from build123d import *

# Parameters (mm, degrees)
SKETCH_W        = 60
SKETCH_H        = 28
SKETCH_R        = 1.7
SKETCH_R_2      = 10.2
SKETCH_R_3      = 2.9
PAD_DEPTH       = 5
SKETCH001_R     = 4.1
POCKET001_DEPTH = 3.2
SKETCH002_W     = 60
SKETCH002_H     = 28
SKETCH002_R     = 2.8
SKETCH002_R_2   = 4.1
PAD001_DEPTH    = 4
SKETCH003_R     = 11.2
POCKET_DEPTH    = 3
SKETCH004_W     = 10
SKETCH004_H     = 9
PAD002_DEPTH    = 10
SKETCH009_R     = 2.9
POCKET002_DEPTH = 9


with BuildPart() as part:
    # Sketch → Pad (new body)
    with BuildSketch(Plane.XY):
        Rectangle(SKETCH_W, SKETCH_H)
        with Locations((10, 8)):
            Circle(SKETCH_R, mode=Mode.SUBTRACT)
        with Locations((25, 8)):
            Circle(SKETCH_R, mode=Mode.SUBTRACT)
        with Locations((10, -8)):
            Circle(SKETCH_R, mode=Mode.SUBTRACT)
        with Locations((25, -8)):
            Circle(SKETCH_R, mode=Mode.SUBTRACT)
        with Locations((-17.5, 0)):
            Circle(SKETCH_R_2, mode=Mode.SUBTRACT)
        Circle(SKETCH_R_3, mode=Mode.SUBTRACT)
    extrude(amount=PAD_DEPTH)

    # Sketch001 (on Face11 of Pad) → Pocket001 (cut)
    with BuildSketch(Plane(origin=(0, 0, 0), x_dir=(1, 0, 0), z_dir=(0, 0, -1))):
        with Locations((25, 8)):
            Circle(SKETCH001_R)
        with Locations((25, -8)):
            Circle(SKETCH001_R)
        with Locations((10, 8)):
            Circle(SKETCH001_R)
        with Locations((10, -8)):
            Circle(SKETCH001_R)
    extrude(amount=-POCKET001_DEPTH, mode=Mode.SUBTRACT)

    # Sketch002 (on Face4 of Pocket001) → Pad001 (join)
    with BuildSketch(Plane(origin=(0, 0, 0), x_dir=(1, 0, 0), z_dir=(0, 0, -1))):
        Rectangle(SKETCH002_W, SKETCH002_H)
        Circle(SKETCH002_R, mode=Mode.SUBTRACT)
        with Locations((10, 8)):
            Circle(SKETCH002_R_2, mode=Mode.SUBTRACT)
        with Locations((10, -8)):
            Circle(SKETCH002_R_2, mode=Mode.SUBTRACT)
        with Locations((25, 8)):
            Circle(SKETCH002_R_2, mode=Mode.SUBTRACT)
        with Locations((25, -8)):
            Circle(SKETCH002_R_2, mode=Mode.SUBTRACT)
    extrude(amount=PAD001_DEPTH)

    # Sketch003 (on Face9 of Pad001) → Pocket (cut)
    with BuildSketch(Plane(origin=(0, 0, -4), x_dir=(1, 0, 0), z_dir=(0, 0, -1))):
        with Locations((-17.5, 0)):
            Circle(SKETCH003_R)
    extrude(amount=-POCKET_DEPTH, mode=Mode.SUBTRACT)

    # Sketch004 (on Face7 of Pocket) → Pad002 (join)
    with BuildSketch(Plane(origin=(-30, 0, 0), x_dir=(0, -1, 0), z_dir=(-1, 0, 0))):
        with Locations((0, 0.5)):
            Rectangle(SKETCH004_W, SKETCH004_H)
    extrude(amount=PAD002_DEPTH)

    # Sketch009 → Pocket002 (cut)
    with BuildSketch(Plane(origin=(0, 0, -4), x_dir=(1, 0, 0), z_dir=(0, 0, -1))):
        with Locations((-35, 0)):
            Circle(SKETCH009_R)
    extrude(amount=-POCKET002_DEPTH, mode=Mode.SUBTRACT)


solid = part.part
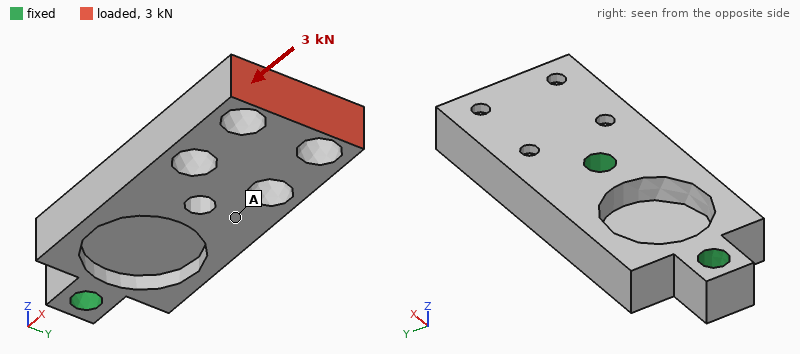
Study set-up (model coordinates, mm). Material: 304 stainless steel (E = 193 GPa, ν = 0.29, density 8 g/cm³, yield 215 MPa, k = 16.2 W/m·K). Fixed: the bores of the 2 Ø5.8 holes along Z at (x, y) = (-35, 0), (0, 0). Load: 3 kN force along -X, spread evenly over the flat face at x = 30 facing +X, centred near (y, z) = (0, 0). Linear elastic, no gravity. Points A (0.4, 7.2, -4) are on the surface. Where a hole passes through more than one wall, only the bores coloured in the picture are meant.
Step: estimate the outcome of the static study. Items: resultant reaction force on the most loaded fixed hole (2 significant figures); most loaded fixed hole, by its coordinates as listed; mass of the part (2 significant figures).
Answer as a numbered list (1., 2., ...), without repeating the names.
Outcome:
1. 2.7 kN
2. (0, 0)
3. 89 g
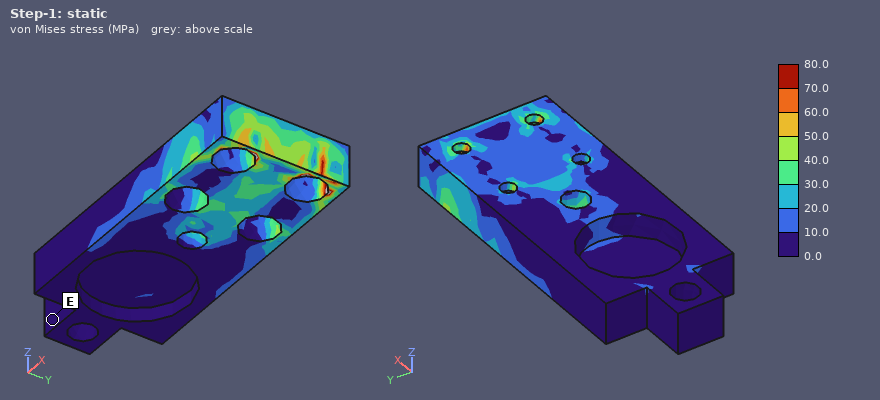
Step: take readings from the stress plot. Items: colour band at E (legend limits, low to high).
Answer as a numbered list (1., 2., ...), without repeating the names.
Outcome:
1. 0.0 to 10.0 MPa
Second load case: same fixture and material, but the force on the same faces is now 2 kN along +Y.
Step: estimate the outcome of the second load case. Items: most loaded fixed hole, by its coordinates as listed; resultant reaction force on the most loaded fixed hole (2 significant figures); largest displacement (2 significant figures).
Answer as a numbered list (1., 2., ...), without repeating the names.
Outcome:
1. (0, 0)
2. 3.0 kN
3. 36 µm
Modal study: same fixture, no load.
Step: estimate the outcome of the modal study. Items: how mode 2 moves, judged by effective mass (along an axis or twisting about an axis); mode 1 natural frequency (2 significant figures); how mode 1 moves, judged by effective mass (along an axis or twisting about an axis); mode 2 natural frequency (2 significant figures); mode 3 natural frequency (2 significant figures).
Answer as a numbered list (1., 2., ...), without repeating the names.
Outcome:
1. along Y
2. 6300 Hz
3. along Z
4. 10 kHz
5. 12 kHz
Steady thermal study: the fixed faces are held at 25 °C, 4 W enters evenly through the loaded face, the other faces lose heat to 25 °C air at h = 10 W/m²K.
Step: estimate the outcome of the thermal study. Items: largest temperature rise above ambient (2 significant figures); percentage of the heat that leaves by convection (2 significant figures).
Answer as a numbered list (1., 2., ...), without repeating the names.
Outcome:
1. 46 K
2. 17 %
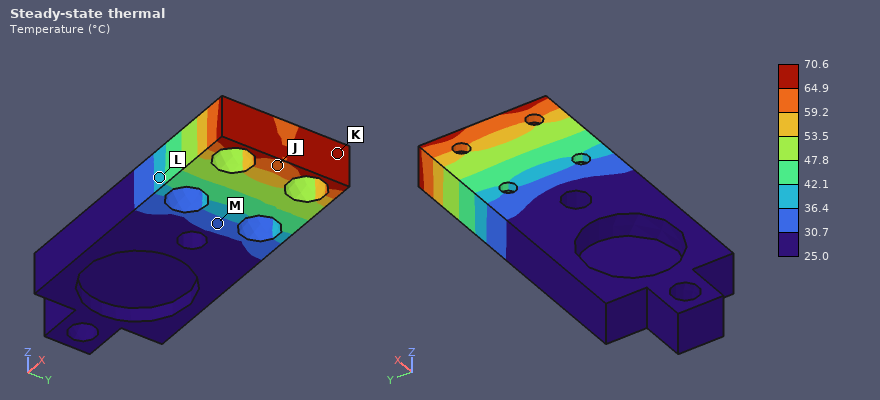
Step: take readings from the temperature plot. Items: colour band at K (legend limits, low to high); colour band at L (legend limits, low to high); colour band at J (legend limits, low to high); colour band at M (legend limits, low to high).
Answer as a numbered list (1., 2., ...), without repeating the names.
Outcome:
1. 64.9 to 70.6 °C
2. 36.4 to 42.1 °C
3. 59.2 to 64.9 °C
4. 30.7 to 36.4 °C
